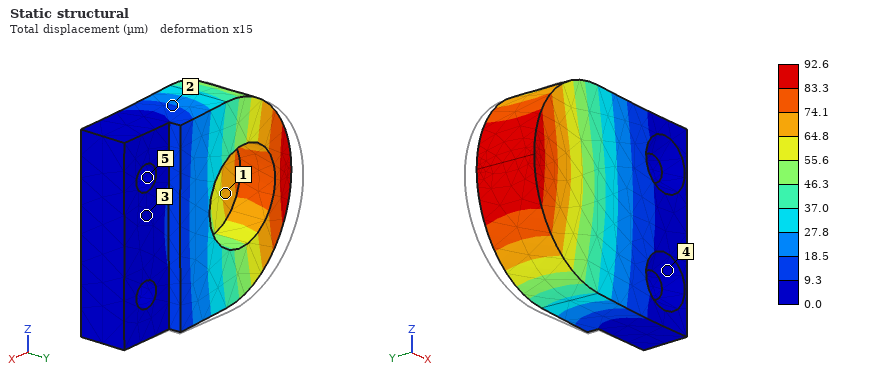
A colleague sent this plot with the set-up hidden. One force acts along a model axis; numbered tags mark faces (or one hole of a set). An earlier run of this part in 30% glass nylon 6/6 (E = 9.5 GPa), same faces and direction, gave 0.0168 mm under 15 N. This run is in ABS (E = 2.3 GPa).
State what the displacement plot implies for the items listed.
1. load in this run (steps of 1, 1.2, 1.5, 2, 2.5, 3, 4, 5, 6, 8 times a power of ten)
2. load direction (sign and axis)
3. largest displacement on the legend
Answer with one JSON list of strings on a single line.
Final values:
["20 N", "-Y", "92.6 µm"]
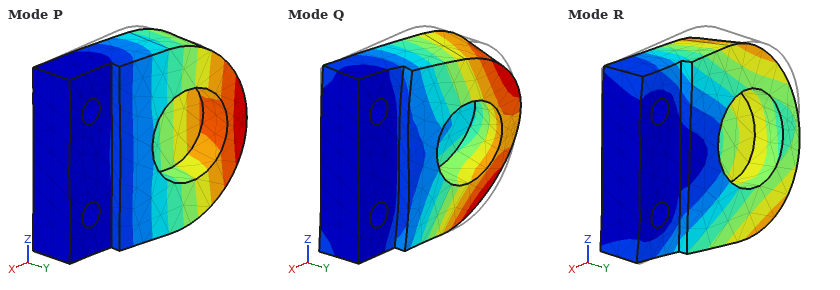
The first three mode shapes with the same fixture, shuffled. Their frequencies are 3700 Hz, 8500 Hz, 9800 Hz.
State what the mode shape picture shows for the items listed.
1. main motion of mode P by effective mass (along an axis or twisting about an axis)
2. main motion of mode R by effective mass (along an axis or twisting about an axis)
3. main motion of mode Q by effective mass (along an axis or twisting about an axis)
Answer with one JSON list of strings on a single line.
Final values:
["along Y", "along Z", "along Z"]
